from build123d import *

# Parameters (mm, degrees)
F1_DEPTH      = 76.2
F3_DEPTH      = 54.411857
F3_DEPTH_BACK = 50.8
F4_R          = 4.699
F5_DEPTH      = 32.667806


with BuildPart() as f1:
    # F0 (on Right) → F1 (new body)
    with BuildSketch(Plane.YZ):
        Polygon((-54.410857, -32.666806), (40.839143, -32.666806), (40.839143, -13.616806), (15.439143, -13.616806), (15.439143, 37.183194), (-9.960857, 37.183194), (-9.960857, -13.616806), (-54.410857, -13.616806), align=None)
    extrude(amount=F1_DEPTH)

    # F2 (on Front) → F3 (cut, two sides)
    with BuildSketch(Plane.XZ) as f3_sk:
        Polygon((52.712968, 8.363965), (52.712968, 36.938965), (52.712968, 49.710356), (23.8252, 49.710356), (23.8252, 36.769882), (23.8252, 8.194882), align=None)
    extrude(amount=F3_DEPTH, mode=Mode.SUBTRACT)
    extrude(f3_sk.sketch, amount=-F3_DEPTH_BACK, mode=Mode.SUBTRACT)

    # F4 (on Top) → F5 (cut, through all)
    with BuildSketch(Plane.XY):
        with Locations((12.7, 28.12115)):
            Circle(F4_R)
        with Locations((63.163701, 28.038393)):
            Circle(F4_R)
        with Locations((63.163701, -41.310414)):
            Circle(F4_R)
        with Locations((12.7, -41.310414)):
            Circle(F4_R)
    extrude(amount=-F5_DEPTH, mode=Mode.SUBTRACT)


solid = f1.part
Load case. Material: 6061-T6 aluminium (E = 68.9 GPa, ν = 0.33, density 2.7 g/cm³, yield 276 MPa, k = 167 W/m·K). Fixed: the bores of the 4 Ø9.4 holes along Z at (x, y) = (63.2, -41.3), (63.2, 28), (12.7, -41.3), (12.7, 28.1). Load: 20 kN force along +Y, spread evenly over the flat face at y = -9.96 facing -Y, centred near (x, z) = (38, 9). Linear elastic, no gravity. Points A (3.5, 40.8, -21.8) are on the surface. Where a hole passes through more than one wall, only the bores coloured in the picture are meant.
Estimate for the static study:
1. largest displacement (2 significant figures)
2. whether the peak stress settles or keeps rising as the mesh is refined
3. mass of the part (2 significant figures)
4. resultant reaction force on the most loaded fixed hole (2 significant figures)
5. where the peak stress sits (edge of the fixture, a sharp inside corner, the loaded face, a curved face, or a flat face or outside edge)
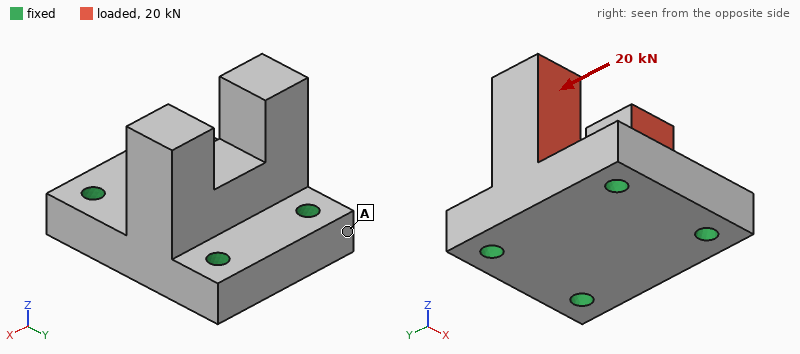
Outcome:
0.12 mm
keeps rising
570 g
8.2 kN
edge of the fixture
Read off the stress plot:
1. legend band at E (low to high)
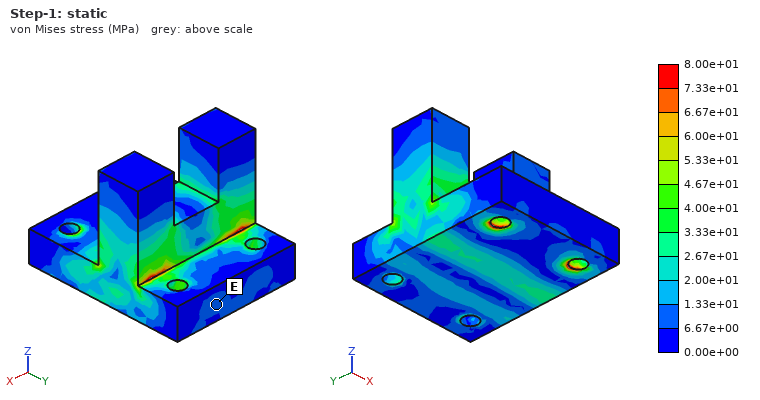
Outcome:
6.67e+00 to 1.33e+01 MPa
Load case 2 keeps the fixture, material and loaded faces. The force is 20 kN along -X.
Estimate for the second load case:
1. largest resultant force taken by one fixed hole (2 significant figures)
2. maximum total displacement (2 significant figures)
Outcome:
11 kN
0.11 mm
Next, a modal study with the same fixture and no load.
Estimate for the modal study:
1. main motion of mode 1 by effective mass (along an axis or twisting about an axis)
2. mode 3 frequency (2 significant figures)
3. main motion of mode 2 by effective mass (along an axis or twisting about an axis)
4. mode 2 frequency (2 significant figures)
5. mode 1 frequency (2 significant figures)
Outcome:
along Y
6800 Hz
along X
6000 Hz
5500 Hz
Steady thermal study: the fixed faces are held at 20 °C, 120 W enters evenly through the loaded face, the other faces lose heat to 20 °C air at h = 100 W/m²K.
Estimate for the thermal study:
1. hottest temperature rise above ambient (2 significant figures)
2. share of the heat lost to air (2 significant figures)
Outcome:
18 K
13 %
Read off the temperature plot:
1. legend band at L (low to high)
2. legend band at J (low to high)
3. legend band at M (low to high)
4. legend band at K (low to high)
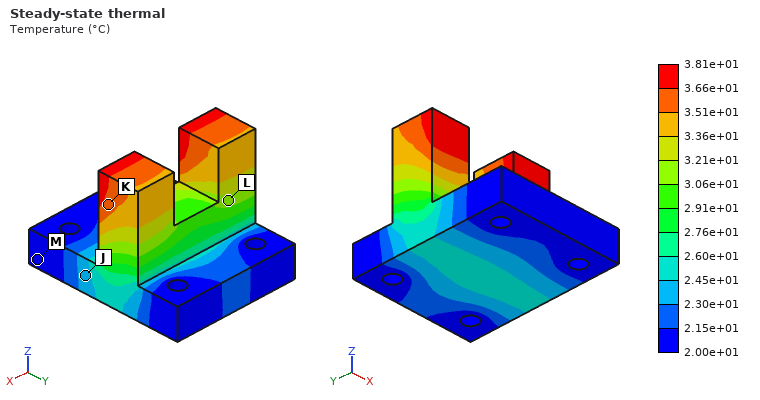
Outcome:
3.06e+01 to 3.21e+01 °C
2.30e+01 to 2.45e+01 °C
2.00e+01 to 2.15e+01 °C
3.51e+01 to 3.66e+01 °C
